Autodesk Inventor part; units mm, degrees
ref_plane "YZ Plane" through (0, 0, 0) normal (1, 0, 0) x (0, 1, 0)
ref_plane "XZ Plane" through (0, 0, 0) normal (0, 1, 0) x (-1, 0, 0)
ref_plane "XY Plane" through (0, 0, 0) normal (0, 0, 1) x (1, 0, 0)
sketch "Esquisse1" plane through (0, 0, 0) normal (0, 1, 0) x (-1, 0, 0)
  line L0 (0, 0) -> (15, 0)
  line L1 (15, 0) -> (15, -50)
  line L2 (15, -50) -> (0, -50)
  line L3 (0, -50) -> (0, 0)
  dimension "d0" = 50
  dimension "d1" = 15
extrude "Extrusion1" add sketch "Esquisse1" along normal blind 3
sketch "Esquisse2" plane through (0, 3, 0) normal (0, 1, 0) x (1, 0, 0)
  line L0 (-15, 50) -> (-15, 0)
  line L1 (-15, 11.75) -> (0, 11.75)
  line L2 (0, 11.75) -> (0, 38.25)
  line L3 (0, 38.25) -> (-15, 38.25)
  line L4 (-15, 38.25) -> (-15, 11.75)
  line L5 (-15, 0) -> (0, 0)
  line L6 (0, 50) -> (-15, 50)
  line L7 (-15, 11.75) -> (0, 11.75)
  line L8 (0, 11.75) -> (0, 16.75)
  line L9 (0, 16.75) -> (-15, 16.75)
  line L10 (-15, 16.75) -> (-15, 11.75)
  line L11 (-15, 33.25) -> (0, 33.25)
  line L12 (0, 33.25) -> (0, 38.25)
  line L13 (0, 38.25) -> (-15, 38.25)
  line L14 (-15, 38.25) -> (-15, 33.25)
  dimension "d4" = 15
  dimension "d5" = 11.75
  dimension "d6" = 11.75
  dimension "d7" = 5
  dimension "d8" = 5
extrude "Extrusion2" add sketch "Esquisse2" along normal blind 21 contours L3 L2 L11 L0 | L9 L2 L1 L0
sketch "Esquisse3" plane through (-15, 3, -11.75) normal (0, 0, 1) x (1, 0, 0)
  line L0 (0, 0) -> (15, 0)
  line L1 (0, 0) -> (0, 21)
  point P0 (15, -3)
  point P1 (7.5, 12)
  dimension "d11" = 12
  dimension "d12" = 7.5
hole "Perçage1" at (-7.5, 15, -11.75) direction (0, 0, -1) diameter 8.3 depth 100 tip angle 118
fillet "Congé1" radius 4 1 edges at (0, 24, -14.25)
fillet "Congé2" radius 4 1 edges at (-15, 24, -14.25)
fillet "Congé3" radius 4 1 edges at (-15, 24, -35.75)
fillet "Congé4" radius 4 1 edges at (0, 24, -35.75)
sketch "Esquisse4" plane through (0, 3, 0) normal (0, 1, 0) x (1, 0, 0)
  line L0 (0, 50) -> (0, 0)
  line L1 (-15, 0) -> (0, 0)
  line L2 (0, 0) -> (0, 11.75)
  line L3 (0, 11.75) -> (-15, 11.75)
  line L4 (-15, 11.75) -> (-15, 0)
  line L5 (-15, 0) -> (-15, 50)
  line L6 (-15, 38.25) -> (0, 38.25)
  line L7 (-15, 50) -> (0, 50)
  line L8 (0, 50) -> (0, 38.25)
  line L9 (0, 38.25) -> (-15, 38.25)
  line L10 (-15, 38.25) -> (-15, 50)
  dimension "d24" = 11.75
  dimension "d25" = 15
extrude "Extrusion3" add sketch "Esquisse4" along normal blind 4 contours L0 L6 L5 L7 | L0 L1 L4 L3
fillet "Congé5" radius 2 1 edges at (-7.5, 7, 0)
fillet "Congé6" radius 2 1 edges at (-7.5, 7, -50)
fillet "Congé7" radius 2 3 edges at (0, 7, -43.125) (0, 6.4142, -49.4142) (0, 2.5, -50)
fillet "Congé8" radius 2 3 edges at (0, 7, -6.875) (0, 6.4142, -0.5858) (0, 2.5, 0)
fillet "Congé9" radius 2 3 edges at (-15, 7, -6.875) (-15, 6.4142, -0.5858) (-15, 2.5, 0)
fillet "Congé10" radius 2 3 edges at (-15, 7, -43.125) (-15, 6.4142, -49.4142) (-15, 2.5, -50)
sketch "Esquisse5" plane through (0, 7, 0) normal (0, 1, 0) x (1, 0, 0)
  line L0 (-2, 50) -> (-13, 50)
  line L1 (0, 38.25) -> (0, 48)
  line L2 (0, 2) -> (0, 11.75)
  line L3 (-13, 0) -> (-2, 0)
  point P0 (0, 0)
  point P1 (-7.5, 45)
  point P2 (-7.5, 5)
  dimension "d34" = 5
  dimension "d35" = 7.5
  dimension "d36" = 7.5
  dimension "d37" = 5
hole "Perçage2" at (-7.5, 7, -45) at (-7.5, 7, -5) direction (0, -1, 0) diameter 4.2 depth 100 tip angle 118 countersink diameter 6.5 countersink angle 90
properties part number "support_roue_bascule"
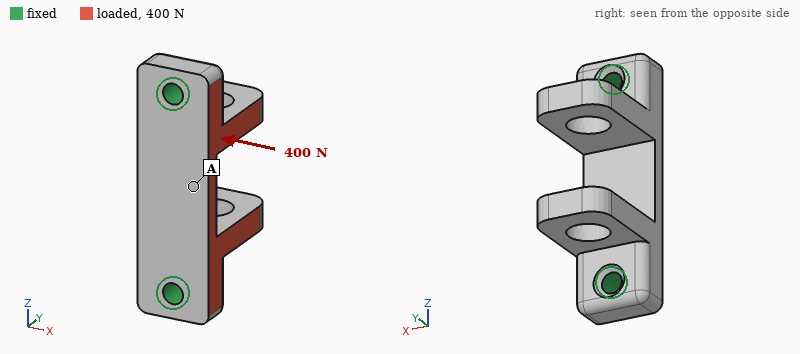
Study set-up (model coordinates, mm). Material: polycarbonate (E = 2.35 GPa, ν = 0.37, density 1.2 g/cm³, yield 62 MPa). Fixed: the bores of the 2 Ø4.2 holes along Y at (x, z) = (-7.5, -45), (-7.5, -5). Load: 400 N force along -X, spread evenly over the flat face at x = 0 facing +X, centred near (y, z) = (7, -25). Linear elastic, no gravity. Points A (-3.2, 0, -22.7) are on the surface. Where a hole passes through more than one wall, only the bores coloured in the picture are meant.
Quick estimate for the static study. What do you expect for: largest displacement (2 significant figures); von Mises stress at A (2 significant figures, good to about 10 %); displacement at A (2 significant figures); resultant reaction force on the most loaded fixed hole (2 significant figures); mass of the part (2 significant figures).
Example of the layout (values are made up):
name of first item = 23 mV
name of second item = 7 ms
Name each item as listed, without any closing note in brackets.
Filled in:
largest displacement = 0.20 mm
von Mises stress at A = 2.9 MPa
displacement at A = 0.050 mm
resultant reaction force on the most loaded fixed hole = 200 N
mass of the part = 7.1 g
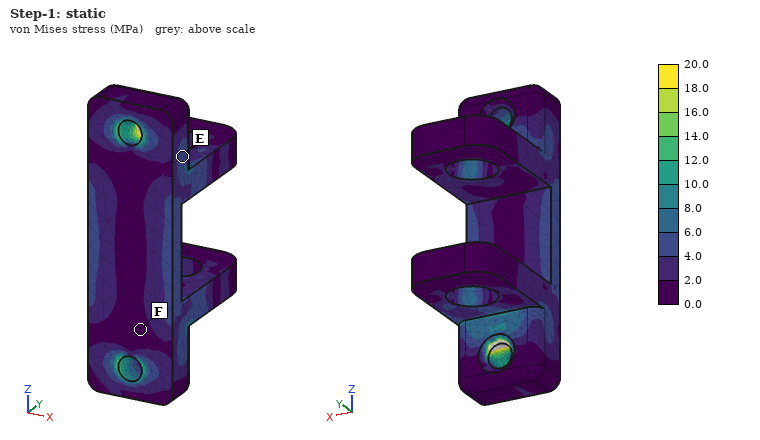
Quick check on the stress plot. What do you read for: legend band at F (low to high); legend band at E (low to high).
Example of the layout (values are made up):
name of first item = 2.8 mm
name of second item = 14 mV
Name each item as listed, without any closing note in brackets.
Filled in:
legend band at F = 0.0 to 2.0 MPa
legend band at E = 4.0 to 6.0 MPa
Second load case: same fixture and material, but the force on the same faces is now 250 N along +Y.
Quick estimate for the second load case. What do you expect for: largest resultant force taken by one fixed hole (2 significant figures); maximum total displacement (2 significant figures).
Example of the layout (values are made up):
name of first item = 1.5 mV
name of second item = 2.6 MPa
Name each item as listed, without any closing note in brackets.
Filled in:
largest resultant force taken by one fixed hole = 130 N
maximum total displacement = 0.20 mm
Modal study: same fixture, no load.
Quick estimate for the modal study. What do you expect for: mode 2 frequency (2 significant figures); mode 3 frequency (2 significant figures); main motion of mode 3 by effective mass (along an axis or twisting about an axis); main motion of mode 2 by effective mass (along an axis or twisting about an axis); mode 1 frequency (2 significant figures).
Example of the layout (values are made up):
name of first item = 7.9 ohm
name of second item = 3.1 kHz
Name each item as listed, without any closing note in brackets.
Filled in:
mode 2 frequency = 2400 Hz
mode 3 frequency = 3000 Hz
main motion of mode 3 by effective mass = along X
main motion of mode 2 by effective mass = along Z
mode 1 frequency = 2300 Hz
